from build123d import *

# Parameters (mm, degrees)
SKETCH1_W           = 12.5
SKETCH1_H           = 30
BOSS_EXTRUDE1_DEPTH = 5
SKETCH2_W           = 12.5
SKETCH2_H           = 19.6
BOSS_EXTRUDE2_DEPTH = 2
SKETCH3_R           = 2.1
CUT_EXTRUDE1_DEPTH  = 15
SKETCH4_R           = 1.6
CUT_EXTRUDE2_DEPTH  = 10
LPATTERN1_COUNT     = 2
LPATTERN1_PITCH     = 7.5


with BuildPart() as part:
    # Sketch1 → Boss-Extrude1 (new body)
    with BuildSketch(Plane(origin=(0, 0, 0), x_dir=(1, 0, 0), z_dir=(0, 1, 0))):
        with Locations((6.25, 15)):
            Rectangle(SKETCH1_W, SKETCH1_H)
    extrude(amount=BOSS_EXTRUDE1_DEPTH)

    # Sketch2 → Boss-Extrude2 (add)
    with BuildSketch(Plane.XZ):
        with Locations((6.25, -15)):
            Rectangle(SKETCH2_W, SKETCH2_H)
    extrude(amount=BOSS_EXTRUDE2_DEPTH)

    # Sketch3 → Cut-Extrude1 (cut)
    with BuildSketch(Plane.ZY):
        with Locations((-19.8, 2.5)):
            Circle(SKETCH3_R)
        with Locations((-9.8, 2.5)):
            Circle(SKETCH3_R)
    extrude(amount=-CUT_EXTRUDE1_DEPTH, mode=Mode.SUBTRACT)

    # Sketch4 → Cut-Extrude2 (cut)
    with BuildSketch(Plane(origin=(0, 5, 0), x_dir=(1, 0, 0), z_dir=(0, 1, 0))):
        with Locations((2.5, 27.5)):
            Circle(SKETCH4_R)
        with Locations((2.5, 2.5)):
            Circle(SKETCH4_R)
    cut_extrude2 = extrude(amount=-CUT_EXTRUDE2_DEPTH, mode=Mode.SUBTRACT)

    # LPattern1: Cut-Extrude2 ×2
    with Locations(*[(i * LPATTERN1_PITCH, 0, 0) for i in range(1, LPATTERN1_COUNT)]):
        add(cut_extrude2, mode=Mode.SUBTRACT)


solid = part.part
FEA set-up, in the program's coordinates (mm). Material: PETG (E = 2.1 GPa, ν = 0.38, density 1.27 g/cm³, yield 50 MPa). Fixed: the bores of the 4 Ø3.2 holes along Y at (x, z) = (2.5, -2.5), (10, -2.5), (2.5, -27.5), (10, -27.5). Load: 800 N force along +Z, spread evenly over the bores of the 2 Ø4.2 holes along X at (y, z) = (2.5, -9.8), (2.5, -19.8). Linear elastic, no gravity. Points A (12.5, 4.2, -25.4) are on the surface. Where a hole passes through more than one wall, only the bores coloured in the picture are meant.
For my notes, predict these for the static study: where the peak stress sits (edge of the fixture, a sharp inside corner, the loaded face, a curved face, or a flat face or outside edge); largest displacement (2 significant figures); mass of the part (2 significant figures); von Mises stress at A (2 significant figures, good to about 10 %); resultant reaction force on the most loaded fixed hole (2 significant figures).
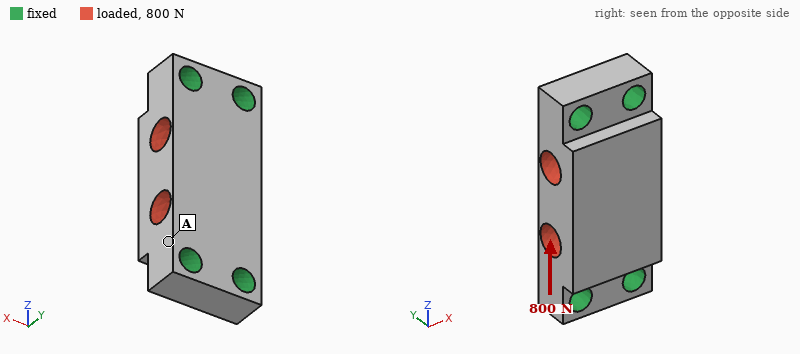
the loaded face
48 µm
2.4 g
4.2 MPa
210 N
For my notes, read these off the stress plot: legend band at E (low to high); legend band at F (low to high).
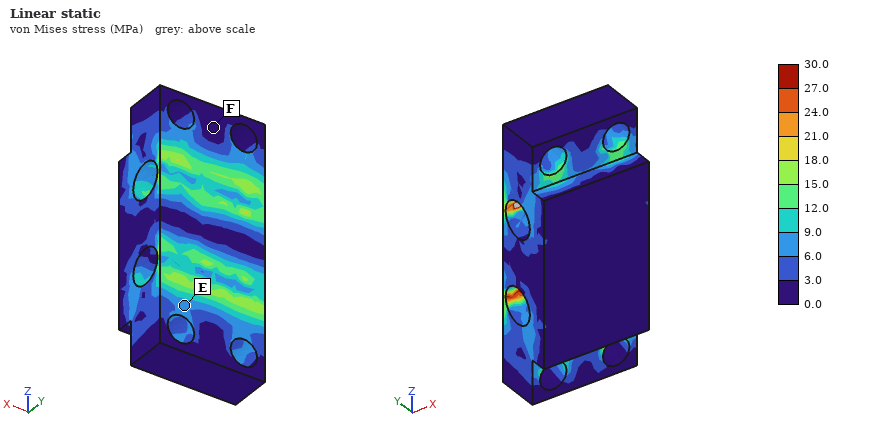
6.0 to 9.0 MPa
0.0 to 3.0 MPa
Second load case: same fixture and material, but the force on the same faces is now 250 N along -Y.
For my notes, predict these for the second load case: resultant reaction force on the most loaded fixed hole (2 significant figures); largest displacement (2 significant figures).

68 N
63 µm
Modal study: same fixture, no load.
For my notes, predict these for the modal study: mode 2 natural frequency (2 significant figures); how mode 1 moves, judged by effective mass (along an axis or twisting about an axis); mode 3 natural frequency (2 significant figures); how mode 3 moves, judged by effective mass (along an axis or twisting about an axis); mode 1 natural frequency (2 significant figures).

11 kHz
along Y
12 kHz
along X
8500 Hz
